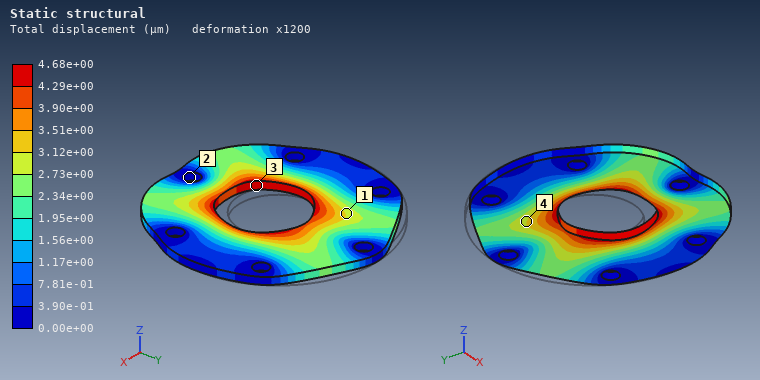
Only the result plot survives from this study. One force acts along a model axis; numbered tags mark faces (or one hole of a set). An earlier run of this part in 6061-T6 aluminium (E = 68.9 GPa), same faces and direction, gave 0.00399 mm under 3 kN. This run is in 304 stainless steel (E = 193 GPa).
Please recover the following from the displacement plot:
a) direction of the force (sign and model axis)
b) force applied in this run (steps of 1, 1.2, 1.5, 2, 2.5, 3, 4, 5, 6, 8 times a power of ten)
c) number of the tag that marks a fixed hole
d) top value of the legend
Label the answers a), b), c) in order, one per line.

a) -Y
b) 10 kN
c) 2
d) 4.68e+00 µm
